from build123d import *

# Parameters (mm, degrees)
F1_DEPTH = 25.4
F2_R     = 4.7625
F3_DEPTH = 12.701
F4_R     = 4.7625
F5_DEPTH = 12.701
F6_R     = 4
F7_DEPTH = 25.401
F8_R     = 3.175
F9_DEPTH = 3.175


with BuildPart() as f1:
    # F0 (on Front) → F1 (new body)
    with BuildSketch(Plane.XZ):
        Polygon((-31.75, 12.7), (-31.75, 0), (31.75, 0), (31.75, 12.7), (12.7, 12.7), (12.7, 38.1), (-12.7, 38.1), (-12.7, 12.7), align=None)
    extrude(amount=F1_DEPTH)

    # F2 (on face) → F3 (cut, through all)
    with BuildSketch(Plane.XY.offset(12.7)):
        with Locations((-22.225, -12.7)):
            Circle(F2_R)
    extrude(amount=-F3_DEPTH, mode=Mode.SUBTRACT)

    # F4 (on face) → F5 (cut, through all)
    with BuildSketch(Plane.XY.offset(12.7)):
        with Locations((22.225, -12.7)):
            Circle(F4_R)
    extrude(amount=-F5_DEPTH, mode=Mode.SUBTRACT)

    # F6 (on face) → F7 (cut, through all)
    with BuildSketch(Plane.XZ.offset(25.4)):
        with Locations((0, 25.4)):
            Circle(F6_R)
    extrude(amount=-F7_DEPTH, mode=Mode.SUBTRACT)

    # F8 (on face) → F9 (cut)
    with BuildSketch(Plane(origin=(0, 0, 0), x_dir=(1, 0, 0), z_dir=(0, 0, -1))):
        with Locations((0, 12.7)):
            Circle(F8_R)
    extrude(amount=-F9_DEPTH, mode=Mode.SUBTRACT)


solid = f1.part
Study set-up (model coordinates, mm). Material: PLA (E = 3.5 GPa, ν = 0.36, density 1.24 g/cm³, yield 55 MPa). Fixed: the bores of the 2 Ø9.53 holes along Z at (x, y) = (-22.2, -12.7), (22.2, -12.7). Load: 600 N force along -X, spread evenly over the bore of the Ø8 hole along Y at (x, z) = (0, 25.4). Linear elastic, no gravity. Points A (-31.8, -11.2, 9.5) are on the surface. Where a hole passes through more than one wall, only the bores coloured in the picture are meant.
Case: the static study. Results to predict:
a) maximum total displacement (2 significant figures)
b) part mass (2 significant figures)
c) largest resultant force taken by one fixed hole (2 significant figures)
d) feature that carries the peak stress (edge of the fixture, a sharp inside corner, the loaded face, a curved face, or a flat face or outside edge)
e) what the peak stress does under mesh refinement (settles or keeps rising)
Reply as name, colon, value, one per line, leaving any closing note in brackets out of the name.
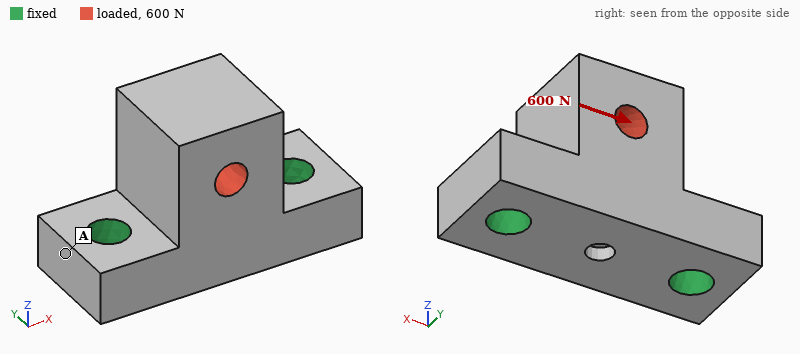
maximum total displacement: 52 µm
part mass: 42 g
largest resultant force taken by one fixed hole: 440 N
feature that carries the peak stress: a sharp inside corner
what the peak stress does under mesh refinement: keeps rising
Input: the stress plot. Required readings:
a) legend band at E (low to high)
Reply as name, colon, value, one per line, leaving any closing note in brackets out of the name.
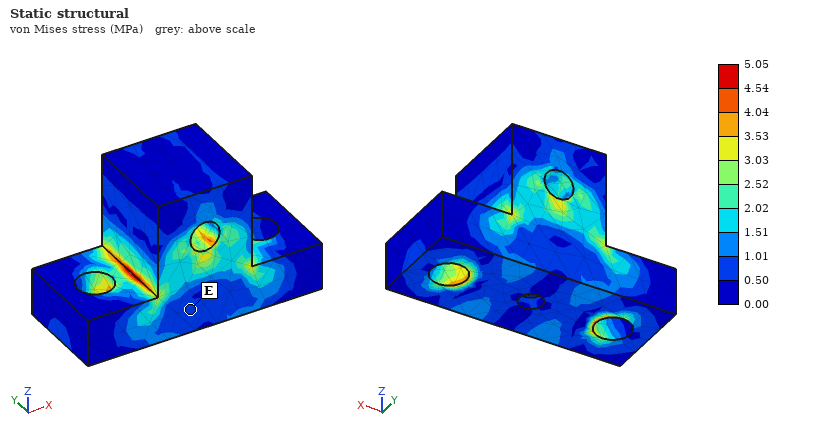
legend band at E: 0.50 to 1.01 MPa
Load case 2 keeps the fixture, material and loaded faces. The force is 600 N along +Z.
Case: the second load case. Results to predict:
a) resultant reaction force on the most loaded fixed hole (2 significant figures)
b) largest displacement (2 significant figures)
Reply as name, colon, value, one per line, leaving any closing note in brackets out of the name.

resultant reaction force on the most loaded fixed hole: 320 N
largest displacement: 19 µm
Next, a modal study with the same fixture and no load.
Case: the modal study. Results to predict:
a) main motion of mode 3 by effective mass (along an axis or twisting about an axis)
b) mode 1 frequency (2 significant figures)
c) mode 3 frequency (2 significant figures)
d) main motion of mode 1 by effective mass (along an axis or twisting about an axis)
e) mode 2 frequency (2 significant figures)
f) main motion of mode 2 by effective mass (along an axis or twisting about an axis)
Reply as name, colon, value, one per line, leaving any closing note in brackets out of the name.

main motion of mode 3 by effective mass: along Z
mode 1 frequency: 2600 Hz
mode 3 frequency: 6100 Hz
main motion of mode 1 by effective mass: along Y
mode 2 frequency: 4400 Hz
main motion of mode 2 by effective mass: along X
